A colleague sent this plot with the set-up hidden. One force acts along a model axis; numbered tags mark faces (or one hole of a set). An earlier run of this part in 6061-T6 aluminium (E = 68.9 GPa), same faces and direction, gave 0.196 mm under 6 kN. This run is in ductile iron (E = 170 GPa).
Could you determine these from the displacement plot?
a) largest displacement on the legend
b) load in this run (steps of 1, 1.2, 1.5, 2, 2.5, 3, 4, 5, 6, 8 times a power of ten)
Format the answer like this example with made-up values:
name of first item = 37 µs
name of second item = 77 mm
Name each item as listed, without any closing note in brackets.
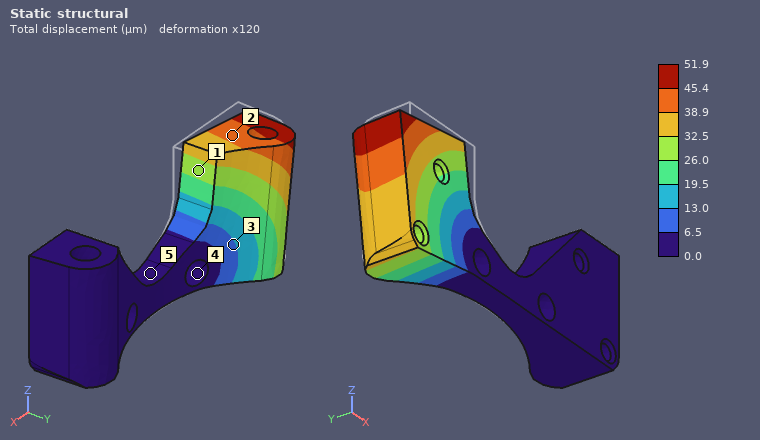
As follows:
largest displacement on the legend = 51.9 µm
load in this run = 4 kN
